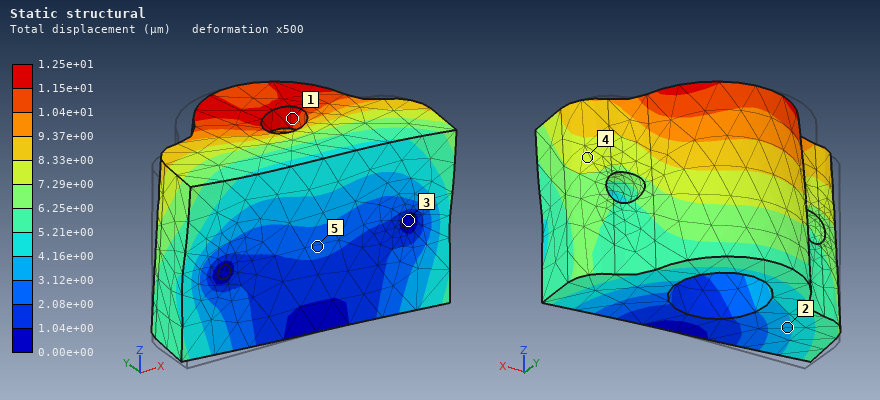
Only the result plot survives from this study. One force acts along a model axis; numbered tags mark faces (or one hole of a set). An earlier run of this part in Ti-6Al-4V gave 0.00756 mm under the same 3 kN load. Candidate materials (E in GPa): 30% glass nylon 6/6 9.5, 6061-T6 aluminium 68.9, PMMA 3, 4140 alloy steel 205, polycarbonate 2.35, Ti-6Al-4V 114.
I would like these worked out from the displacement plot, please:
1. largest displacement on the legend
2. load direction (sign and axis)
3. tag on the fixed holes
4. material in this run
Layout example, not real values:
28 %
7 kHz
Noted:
1.25e+01 µm
+X
3
6061-T6 aluminium
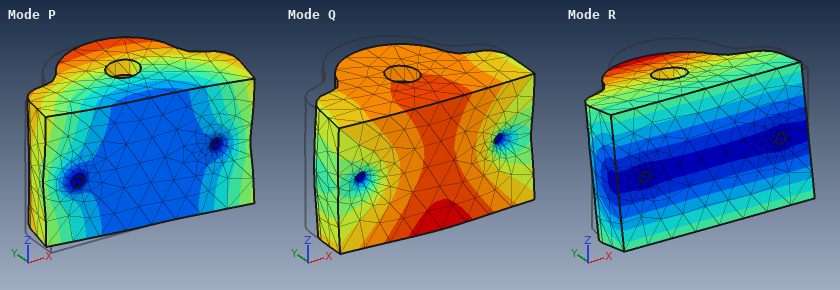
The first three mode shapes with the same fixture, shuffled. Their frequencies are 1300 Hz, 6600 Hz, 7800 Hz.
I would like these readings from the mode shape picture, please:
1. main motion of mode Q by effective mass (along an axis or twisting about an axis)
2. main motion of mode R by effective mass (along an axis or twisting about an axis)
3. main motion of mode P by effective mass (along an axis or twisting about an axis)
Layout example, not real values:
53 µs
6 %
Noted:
along Y
along Z
along X
